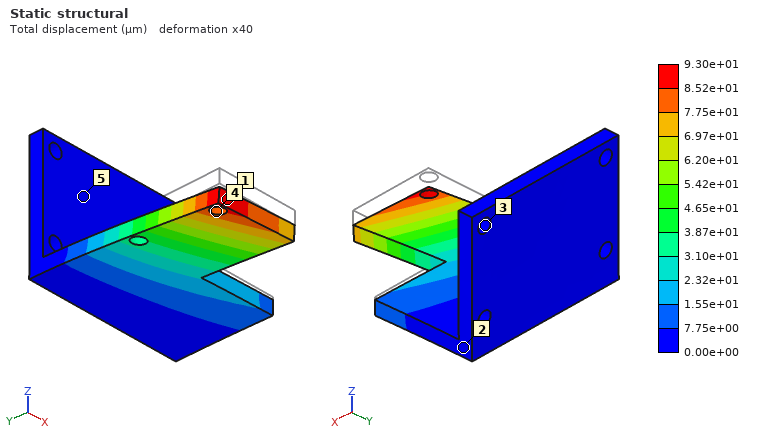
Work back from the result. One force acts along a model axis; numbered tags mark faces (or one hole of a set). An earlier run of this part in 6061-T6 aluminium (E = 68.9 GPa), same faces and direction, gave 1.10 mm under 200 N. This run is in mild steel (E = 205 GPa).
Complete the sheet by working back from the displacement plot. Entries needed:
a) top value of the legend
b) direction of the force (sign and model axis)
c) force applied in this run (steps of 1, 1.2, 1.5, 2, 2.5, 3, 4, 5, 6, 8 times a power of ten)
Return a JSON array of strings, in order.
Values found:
["9.30e+01 µm", "-Z", "50 N"]
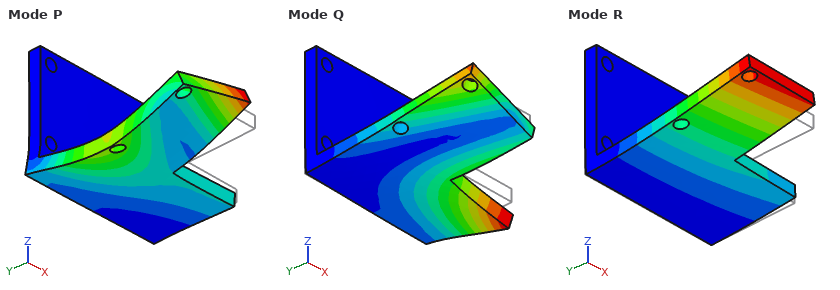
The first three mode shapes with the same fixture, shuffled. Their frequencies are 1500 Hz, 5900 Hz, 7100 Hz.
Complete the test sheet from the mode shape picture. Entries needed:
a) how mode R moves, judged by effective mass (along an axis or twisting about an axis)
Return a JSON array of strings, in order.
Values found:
["along Z"]
